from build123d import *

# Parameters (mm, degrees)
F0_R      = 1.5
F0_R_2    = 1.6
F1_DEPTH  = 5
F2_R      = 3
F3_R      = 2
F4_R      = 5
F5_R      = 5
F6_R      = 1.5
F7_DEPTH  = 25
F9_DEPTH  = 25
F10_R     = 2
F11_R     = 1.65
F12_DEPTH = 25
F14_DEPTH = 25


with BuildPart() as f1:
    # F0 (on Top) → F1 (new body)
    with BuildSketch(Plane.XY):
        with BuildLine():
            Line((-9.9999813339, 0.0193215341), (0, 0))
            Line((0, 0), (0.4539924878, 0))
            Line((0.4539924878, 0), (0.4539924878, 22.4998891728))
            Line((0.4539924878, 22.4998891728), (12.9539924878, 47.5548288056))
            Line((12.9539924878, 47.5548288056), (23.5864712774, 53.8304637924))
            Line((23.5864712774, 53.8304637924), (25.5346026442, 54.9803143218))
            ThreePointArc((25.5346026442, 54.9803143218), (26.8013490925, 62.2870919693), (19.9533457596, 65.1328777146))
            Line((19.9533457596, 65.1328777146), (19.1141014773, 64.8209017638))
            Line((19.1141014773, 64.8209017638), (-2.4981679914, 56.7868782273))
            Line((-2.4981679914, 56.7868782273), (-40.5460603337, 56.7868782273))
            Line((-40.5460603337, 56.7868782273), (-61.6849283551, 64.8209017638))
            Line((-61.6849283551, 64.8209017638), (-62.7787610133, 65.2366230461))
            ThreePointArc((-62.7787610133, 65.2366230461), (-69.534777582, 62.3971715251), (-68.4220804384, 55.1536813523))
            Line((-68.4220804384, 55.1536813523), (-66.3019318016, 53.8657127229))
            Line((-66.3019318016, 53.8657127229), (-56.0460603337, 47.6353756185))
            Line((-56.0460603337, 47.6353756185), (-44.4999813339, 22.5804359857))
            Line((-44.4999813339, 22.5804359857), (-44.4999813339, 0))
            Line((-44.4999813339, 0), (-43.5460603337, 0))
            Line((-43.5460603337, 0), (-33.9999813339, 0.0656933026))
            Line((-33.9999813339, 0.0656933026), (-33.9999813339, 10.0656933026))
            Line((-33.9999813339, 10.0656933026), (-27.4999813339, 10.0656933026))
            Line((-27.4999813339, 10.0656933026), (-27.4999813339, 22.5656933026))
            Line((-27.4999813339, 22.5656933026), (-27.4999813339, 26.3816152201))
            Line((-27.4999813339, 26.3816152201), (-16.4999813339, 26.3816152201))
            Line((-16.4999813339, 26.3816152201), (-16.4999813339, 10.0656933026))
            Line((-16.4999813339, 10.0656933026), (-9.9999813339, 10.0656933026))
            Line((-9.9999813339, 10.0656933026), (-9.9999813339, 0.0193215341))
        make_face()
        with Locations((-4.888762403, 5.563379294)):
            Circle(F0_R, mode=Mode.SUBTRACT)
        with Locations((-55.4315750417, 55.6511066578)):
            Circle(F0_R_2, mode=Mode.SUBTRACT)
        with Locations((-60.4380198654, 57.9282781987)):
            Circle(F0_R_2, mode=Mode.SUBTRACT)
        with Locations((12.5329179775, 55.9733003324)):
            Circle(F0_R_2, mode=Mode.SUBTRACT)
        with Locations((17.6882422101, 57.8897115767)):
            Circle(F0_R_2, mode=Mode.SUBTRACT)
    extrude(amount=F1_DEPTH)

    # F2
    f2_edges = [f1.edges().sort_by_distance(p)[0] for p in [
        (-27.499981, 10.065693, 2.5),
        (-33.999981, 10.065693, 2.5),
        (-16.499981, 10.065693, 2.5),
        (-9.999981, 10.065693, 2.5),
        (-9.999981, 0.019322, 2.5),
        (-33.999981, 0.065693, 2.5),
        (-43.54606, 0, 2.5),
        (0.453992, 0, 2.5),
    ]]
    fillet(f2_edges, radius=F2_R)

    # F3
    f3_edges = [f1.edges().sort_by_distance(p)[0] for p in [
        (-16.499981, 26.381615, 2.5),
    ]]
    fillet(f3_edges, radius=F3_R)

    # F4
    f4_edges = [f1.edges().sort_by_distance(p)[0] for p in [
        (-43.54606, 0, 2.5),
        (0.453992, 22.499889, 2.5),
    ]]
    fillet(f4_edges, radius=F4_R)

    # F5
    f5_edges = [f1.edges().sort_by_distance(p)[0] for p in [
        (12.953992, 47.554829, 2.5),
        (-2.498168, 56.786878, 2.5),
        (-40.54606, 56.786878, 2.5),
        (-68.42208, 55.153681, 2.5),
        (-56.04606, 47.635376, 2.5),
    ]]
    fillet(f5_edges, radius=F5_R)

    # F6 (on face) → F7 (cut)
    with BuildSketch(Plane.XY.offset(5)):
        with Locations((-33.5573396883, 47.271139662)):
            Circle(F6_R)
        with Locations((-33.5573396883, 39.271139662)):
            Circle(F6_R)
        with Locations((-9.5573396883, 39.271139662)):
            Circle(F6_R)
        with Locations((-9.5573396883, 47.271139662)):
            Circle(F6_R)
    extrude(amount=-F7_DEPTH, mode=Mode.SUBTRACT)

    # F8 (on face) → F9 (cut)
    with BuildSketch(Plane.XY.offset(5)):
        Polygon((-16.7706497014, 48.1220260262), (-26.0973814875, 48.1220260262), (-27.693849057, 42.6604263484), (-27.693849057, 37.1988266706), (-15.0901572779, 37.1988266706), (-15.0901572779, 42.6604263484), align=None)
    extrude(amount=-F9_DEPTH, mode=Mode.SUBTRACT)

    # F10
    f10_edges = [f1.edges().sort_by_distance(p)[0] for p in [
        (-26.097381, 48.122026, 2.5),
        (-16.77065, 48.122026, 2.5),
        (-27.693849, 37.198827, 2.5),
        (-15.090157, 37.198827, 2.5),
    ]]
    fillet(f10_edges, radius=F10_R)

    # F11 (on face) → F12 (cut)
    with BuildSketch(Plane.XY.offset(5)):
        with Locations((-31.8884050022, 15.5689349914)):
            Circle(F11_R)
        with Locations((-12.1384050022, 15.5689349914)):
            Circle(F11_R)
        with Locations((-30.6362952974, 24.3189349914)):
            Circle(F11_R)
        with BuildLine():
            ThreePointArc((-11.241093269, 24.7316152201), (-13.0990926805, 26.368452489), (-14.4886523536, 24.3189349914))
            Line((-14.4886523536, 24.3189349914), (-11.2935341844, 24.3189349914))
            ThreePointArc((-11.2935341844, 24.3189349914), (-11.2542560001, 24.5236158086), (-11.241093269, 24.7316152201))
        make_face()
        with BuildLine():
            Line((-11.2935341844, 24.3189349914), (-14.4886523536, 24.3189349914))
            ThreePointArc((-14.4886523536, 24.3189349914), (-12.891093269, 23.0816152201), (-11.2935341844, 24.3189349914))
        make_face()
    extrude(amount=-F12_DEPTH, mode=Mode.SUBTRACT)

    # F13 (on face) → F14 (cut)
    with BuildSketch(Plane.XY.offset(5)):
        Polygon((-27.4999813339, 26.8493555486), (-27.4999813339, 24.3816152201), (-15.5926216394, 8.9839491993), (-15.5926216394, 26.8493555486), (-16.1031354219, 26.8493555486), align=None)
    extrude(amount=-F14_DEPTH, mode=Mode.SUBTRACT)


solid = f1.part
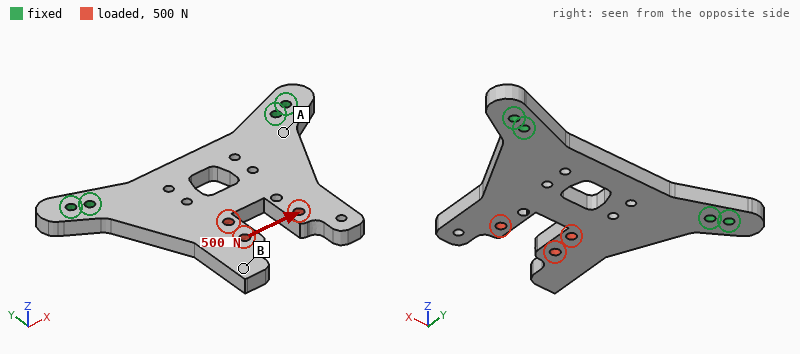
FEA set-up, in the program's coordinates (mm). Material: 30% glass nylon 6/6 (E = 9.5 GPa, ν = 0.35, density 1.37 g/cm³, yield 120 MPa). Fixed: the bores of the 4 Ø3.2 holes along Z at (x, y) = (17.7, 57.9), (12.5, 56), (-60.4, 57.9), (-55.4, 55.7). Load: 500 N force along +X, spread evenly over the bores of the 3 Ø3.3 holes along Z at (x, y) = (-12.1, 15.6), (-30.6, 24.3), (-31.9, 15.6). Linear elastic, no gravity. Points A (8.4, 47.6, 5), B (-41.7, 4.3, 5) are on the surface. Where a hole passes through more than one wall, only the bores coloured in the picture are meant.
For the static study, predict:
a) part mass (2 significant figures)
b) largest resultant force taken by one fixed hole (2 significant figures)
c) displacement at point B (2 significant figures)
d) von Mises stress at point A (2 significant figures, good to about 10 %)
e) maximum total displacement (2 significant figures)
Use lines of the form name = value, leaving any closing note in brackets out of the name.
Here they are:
part mass = 19 g
largest resultant force taken by one fixed hole = 270 N
displacement at point B = 89 µm
von Mises stress at point A = 5.9 MPa
maximum total displacement = 99 µm
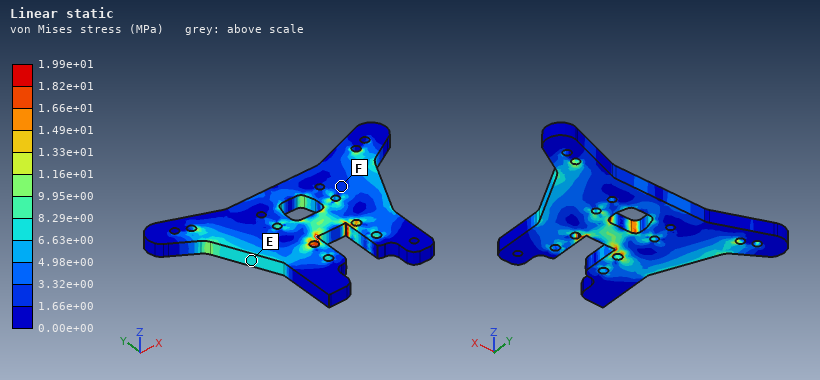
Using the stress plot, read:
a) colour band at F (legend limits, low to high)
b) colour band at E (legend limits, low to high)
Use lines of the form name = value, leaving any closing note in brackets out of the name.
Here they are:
colour band at F = 1.66e+00 to 3.32e+00 MPa
colour band at E = 6.63e+00 to 8.29e+00 MPa
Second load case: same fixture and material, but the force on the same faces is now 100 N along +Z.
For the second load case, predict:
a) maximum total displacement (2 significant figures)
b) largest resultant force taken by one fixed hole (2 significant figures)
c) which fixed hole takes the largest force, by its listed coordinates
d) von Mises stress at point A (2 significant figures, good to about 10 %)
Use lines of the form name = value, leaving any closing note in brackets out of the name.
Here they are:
maximum total displacement = 1.2 mm
largest resultant force taken by one fixed hole = 120 N
which fixed hole takes the largest force, by its listed coordinates = (-55.4, 55.7)
von Mises stress at point A = 22 MPa
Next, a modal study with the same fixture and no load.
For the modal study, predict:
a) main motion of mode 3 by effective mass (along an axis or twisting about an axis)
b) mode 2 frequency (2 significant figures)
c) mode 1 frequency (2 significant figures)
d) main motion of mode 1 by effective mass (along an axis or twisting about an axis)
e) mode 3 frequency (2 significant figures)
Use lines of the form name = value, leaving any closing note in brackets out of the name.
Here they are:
main motion of mode 3 by effective mass = along Z
mode 2 frequency = 1300 Hz
mode 1 frequency = 670 Hz
main motion of mode 1 by effective mass = along Z
mode 3 frequency = 2500 Hz
